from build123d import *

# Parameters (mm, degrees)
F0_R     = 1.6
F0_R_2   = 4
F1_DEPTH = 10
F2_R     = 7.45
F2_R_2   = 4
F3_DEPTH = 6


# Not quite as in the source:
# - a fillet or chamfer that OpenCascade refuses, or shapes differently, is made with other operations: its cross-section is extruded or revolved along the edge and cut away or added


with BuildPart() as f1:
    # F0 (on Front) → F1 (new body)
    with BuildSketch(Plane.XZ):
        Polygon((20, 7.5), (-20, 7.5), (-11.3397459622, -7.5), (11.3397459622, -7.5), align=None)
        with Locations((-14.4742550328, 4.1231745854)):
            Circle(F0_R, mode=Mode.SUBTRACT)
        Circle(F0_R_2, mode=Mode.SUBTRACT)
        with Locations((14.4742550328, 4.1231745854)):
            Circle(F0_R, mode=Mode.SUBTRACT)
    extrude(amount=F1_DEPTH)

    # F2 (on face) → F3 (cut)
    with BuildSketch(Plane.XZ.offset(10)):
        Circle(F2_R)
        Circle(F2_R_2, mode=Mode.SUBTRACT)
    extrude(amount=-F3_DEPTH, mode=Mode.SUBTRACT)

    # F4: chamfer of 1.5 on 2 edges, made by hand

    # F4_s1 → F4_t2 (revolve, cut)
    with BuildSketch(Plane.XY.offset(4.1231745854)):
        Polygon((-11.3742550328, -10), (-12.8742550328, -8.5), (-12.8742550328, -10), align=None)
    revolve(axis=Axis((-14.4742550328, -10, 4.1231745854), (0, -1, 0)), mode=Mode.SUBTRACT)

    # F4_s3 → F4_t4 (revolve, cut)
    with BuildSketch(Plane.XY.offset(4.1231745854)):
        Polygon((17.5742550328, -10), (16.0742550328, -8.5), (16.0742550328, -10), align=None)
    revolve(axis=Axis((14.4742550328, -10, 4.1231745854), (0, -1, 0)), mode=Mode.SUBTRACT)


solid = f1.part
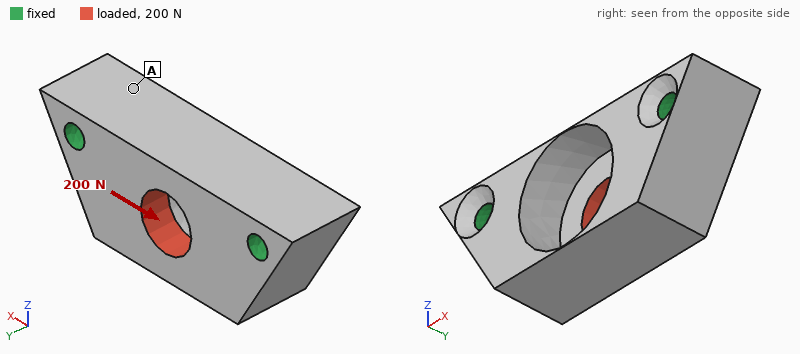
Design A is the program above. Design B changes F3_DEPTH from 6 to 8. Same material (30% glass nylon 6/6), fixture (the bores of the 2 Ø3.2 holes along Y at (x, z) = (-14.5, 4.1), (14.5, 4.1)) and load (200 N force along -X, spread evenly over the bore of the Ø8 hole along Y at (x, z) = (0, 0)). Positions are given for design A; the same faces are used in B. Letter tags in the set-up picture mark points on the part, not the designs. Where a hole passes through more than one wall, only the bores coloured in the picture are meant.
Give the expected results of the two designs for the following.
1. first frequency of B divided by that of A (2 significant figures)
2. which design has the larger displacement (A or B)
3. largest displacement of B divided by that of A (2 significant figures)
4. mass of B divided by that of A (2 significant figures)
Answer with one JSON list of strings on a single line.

["1.1", "B", "1.7", "0.92"]
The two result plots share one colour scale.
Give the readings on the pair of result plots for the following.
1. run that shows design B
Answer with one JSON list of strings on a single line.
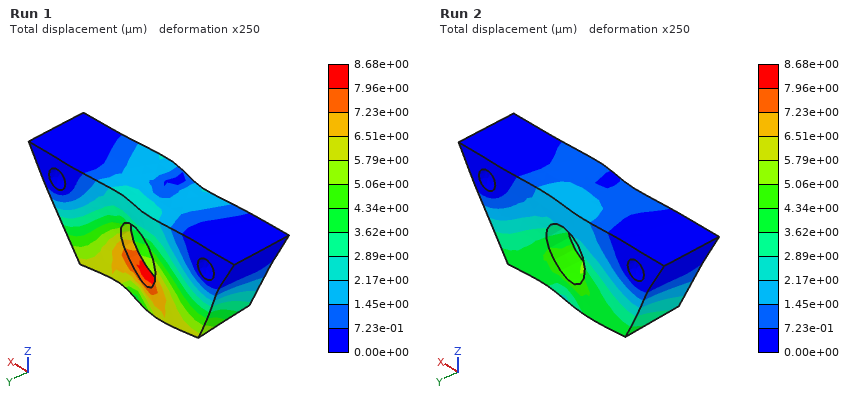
["Run 1"]
